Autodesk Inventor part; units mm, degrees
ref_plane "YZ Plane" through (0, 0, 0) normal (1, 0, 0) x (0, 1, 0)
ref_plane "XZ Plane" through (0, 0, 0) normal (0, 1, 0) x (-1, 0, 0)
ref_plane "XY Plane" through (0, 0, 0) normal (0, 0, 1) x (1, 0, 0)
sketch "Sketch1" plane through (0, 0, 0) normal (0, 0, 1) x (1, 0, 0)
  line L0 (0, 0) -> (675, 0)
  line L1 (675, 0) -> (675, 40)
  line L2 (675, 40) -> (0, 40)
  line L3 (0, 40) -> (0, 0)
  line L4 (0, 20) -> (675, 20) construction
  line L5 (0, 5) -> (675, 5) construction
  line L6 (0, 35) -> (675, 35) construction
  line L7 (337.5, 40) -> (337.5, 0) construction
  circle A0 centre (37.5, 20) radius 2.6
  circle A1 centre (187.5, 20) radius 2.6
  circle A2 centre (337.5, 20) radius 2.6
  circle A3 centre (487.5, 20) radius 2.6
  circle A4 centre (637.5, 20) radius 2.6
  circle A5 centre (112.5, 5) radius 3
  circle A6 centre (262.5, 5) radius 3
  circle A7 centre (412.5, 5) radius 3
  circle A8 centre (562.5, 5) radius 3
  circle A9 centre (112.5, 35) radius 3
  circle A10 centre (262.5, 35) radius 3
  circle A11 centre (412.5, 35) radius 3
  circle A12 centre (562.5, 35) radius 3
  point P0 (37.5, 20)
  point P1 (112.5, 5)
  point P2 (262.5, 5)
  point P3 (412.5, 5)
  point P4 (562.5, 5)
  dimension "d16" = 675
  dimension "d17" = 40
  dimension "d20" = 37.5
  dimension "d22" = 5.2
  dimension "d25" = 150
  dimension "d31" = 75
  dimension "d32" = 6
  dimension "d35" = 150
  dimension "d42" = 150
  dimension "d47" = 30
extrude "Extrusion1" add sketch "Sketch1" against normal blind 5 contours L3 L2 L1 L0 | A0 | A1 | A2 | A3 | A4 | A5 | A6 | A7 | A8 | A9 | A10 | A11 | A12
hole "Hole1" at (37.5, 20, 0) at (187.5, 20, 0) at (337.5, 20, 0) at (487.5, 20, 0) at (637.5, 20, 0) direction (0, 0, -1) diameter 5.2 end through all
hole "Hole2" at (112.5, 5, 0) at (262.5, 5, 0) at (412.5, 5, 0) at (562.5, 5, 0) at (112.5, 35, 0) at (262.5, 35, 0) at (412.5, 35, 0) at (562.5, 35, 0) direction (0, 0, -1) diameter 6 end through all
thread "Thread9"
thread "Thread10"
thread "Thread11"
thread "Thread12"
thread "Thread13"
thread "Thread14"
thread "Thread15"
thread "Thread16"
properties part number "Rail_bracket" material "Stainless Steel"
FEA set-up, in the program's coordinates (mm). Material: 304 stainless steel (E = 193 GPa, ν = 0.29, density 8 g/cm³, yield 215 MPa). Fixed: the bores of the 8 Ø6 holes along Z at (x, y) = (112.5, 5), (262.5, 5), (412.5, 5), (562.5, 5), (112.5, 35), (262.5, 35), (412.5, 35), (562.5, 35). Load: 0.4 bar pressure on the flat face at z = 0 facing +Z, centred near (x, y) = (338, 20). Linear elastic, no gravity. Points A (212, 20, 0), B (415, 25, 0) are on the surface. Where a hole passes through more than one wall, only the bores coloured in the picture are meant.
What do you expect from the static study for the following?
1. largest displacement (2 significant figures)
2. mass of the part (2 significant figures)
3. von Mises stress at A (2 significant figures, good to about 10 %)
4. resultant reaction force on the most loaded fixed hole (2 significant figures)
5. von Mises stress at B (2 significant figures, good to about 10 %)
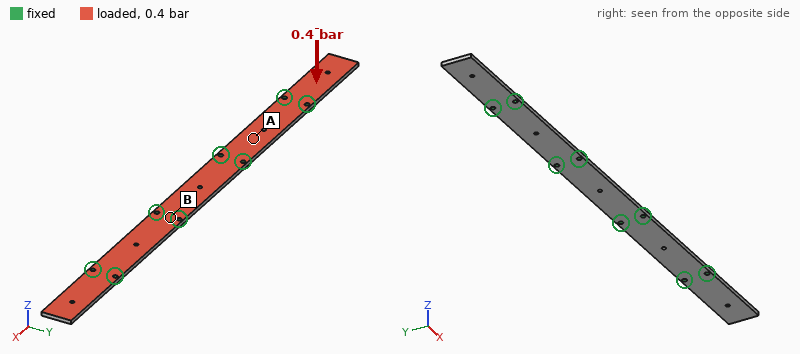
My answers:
0.38 mm
1.1 kg
5.4 MPa
150 N
12 MPa
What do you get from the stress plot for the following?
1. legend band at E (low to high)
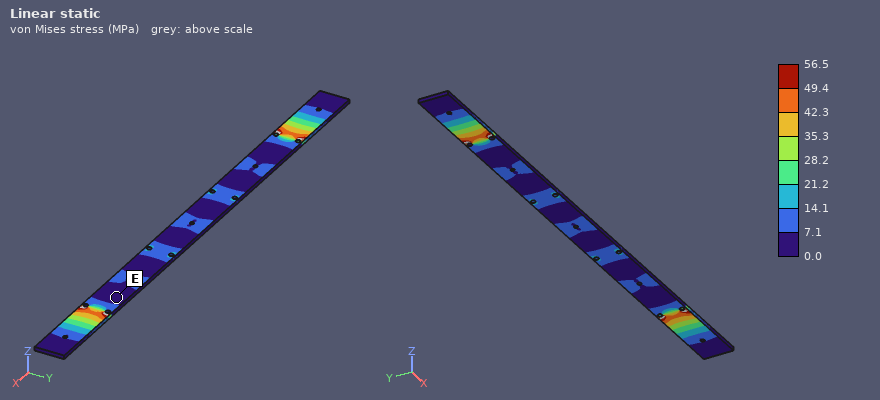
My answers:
0.0 to 7.1 MPa
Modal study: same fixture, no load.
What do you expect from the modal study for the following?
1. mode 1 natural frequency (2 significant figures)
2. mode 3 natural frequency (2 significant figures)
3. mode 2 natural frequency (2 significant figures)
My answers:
320 Hz
1100 Hz
320 Hz
